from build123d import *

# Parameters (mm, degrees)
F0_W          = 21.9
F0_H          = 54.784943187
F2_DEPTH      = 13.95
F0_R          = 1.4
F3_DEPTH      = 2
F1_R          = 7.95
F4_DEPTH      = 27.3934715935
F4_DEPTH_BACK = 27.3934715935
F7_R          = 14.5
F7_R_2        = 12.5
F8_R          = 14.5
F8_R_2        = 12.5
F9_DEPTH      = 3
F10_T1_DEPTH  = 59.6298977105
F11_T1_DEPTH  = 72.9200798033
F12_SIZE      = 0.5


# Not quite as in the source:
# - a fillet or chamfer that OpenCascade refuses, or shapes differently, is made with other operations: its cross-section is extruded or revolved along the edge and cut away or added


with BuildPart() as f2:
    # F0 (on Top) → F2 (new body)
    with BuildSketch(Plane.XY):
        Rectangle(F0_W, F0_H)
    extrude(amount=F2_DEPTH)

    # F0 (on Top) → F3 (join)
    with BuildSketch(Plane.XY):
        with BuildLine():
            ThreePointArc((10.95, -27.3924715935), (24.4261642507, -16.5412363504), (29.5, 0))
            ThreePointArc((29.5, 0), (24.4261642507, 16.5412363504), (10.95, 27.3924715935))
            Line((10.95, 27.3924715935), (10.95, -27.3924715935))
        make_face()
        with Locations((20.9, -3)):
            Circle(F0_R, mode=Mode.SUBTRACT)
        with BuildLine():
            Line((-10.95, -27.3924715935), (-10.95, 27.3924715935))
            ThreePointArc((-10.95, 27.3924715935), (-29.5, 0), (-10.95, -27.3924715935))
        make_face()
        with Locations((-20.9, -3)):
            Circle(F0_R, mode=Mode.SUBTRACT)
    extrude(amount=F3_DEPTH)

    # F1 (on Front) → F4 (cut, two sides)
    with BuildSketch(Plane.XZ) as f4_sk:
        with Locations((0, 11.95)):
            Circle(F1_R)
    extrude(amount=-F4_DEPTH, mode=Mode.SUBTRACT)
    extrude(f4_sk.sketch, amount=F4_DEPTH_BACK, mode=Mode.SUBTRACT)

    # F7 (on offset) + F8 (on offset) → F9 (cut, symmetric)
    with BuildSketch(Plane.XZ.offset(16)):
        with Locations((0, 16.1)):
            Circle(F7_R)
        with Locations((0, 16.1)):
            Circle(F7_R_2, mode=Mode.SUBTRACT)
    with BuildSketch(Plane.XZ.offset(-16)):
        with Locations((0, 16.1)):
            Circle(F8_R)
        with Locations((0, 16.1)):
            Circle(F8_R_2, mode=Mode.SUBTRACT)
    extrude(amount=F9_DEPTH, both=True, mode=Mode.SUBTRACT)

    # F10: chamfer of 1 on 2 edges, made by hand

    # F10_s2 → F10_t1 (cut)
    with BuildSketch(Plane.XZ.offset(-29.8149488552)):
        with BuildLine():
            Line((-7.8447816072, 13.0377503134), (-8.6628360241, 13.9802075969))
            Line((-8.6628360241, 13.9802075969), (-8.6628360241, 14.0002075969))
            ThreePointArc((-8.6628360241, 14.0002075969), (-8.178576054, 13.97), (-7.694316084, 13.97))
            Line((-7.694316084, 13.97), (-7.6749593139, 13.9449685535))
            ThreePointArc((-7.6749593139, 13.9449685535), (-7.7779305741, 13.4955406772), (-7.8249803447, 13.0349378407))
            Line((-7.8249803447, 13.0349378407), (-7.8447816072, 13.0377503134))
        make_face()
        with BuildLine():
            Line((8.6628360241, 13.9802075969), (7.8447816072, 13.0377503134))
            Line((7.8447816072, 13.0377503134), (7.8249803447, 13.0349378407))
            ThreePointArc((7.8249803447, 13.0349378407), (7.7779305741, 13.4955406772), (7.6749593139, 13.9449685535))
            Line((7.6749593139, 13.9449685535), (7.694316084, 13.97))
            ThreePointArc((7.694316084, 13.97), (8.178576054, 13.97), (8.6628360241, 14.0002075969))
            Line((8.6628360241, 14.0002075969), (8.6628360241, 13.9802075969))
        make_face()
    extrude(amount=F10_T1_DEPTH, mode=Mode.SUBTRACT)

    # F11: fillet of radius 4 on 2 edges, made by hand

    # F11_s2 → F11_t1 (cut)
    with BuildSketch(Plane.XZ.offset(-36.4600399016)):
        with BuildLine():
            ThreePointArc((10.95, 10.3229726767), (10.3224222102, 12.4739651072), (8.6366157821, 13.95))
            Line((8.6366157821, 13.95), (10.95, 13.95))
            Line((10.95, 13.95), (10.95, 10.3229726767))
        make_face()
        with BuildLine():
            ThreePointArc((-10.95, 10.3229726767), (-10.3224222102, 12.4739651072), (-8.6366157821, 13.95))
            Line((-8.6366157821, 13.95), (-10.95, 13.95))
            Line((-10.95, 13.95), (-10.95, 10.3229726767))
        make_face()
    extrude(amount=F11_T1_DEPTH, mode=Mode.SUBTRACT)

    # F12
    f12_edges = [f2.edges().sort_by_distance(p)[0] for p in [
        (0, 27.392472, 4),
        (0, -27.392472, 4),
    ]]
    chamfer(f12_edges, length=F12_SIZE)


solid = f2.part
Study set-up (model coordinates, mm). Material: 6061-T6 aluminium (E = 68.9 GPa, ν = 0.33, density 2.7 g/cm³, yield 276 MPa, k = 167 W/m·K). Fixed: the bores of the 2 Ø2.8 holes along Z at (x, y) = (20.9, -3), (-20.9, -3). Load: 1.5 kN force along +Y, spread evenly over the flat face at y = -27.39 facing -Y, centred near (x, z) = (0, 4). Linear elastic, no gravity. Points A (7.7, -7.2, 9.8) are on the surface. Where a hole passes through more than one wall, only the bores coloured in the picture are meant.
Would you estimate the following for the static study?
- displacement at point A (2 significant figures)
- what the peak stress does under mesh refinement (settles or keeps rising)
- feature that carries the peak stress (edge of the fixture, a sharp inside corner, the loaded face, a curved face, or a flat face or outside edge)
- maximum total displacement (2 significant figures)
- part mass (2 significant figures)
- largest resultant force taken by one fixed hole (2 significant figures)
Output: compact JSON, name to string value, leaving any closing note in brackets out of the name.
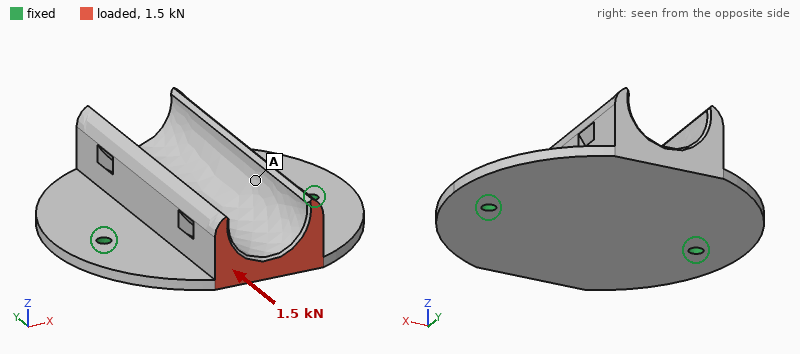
{"displacement at point A": "0.11 mm", "what the peak stress does under mesh refinement": "keeps rising", "feature that carries the peak stress": "edge of the fixture", "maximum total displacement": "0.35 mm", "part mass": "31 g", "largest resultant force taken by one fixed hole": "750 N"}
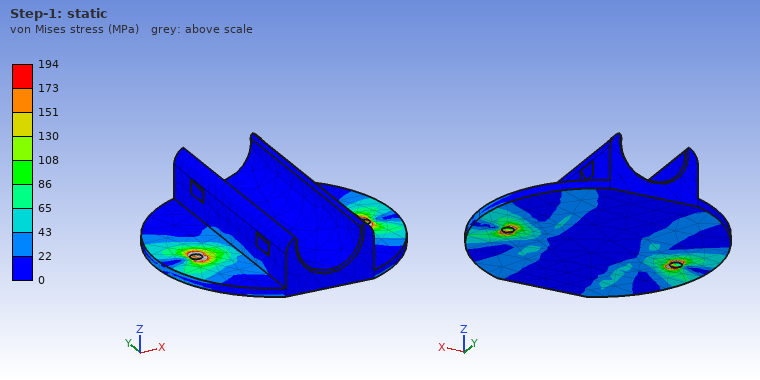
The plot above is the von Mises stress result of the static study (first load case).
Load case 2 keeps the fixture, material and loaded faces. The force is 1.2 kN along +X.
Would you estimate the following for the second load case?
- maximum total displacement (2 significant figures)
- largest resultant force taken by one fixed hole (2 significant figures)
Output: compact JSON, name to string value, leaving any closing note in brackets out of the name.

{"maximum total displacement": "52 µm", "largest resultant force taken by one fixed hole": "920 N"}
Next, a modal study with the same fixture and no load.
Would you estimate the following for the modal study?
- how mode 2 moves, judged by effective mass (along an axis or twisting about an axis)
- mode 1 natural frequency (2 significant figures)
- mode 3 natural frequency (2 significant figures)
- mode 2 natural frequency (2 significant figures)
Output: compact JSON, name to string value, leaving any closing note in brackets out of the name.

{"how mode 2 moves, judged by effective mass": "along Z", "mode 1 natural frequency": "1300 Hz", "mode 3 natural frequency": "5800 Hz", "mode 2 natural frequency": "3500 Hz"}
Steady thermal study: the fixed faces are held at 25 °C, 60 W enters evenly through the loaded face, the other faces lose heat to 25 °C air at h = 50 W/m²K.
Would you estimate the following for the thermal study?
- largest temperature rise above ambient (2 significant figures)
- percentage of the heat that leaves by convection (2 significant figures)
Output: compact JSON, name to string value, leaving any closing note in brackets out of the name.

{"largest temperature rise above ambient": "75 K", "percentage of the heat that leaves by convection": "23 %"}
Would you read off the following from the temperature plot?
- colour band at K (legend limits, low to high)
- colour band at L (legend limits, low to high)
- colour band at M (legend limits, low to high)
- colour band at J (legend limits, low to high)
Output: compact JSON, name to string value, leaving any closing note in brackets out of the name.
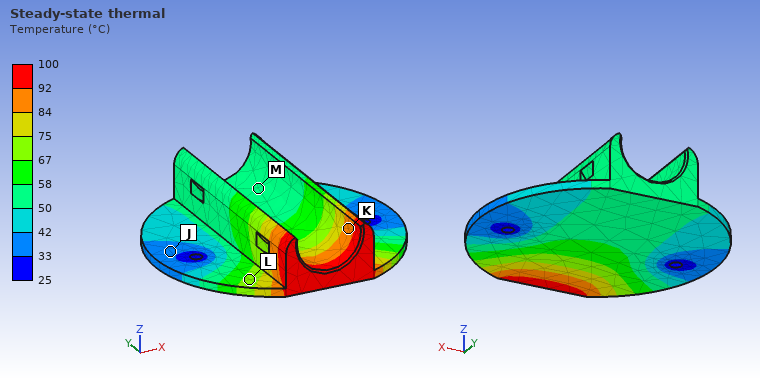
{"colour band at K": "84 to 92 °C", "colour band at L": "67 to 75 °C", "colour band at M": "50 to 58 °C", "colour band at J": "33 to 42 °C"}
